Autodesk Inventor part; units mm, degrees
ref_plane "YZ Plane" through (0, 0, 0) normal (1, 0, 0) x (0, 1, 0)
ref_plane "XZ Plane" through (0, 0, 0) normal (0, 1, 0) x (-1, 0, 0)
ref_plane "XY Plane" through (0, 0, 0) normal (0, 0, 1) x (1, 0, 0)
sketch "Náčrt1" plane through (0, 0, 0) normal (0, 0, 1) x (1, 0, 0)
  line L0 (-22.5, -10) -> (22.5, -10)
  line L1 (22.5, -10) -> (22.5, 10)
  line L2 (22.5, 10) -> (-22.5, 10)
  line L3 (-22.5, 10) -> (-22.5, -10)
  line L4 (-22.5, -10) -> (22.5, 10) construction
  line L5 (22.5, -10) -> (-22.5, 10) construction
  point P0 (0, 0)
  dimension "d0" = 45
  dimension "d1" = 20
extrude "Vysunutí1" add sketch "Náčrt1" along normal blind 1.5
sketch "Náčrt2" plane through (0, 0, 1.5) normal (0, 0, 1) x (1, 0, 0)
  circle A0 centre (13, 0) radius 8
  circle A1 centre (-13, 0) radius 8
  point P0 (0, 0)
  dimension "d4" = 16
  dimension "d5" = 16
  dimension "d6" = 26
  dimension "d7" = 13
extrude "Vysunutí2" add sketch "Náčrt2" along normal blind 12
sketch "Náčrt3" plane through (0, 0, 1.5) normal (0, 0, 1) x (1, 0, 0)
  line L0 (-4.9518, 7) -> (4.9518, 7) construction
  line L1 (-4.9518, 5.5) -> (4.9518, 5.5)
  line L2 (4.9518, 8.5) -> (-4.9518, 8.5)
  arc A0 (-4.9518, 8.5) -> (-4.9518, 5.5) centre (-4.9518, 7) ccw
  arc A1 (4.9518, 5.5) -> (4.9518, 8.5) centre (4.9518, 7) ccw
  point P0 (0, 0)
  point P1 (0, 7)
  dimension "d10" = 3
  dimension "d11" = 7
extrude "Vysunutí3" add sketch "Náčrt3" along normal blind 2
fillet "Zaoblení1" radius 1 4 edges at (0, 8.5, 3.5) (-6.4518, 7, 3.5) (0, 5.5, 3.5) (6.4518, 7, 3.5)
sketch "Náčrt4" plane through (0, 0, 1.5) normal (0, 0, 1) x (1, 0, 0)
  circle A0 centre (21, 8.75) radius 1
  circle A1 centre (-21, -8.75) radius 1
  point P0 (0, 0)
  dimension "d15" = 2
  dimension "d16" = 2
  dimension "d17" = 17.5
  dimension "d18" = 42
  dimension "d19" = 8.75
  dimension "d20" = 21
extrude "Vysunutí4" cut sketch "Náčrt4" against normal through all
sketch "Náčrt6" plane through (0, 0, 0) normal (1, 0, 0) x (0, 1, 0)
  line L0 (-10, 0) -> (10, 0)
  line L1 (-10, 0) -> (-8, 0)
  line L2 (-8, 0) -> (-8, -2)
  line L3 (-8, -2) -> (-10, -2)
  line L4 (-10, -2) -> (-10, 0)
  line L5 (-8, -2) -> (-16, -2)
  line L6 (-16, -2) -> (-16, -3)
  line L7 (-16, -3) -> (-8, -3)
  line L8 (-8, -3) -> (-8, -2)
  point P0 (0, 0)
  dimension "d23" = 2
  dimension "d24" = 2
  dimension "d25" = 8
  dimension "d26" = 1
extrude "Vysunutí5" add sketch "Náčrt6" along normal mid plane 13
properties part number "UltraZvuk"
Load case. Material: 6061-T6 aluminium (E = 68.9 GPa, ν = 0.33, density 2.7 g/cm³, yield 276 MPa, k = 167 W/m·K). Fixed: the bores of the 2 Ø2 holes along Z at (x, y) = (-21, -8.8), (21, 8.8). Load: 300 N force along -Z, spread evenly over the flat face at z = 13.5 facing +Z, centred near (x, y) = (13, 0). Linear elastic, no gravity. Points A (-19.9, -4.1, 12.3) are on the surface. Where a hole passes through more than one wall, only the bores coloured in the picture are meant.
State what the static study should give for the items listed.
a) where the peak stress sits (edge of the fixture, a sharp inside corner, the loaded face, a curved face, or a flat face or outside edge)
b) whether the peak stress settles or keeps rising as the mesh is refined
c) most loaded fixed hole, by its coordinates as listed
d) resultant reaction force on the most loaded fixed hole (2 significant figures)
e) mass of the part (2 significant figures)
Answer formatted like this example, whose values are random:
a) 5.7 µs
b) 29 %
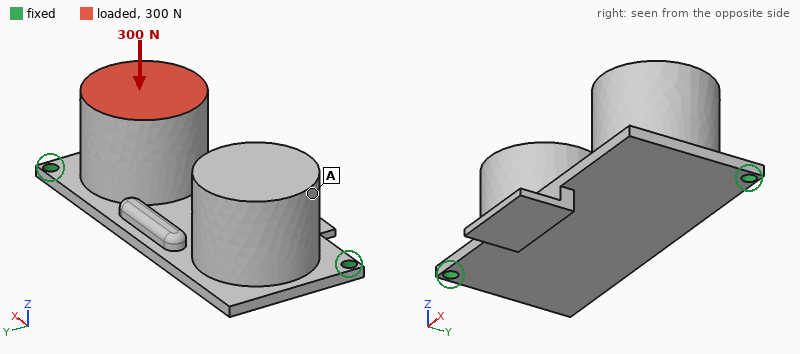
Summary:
a) edge of the fixture
b) keeps rising
c) (21, 8.8)
d) 240 N
e) 17 g
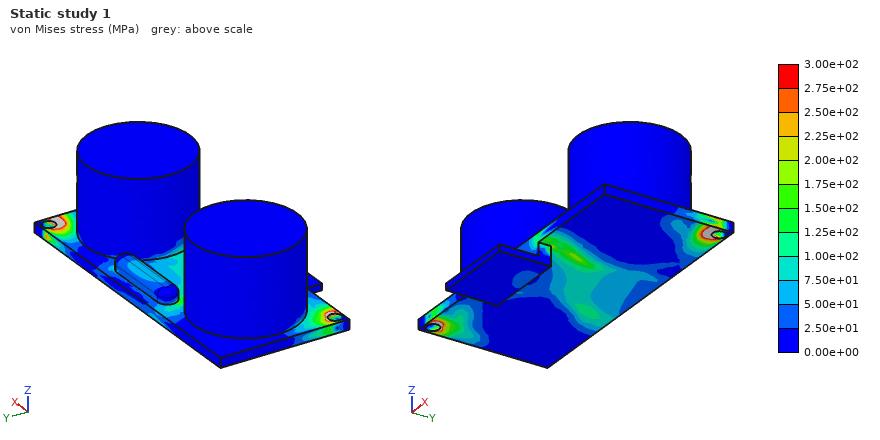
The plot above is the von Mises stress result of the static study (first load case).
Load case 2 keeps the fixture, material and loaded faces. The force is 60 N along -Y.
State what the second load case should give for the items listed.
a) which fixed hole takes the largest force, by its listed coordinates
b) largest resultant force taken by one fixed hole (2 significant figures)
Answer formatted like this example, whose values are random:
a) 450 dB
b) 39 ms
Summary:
a) (21, 8.8)
b) 50 N
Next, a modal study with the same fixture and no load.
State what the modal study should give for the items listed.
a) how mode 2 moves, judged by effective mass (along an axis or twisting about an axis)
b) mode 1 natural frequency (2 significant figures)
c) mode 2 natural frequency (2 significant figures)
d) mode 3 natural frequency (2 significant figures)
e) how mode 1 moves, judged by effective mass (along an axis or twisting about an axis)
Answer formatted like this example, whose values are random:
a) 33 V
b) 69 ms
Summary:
a) along Z
b) 1400 Hz
c) 1800 Hz
d) 3100 Hz
e) along Y
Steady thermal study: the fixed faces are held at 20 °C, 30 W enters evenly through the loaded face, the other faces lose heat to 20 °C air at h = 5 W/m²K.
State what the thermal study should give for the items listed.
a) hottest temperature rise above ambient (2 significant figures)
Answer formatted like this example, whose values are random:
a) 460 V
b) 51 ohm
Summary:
a) 70 K
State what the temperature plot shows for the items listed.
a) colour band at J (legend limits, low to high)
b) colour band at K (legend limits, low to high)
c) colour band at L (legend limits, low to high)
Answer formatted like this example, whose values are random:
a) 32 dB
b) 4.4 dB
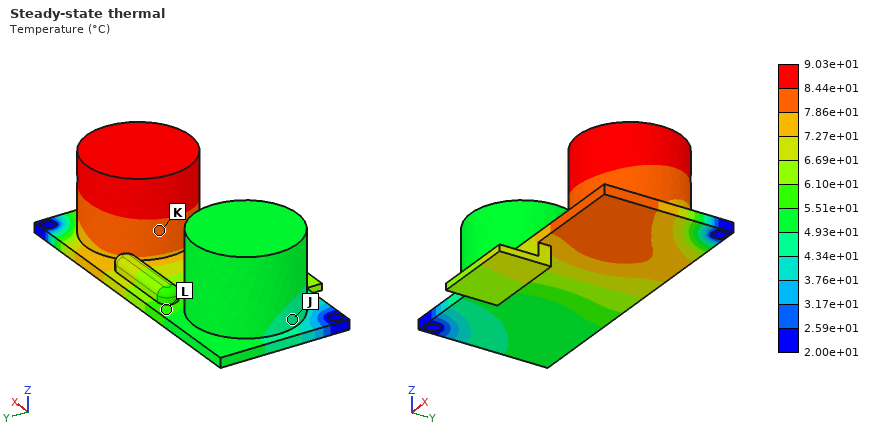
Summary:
a) 4.34e+01 to 4.93e+01 °C
b) 7.86e+01 to 8.44e+01 °C
c) 5.51e+01 to 6.10e+01 °C
